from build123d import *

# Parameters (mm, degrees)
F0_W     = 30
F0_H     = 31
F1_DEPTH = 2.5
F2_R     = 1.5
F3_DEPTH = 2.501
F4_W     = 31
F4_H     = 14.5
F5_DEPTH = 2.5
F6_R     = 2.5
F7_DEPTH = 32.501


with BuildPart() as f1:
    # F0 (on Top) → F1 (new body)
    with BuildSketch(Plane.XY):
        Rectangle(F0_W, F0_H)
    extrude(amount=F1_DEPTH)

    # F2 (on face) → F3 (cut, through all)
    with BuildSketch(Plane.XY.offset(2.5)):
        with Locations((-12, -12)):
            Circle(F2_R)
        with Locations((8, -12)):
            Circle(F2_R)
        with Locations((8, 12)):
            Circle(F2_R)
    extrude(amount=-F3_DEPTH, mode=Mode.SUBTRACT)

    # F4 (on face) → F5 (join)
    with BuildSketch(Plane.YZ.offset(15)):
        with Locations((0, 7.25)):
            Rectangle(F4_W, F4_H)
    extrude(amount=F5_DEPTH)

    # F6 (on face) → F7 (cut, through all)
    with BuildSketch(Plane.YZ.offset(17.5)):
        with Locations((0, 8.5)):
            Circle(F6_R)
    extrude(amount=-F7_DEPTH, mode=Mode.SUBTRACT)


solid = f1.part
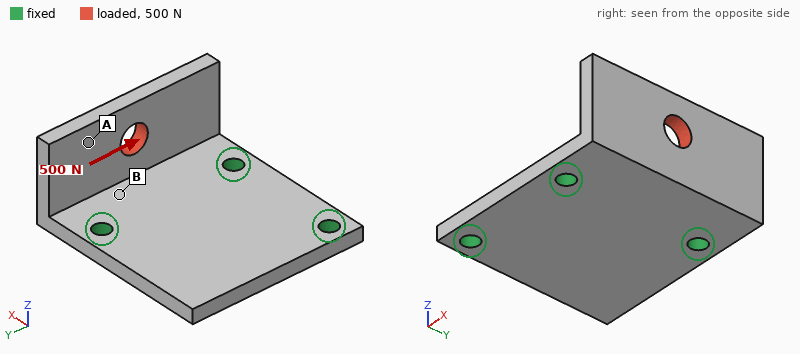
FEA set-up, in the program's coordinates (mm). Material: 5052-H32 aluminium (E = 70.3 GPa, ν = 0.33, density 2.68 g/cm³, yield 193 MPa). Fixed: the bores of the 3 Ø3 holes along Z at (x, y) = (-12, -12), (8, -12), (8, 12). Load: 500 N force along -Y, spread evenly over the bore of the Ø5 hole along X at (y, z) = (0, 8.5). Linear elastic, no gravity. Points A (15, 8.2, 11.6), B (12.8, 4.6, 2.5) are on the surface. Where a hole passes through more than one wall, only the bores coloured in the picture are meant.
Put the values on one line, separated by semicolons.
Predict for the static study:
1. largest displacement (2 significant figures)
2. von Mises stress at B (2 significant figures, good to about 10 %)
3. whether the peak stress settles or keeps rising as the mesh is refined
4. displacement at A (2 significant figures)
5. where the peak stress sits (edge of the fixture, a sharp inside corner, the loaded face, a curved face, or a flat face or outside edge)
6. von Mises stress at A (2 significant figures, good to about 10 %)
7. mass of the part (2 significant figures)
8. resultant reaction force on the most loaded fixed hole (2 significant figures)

35 µm; 33 MPa; keeps rising; 23 µm; edge of the fixture; 12 MPa; 9.0 g; 330 N
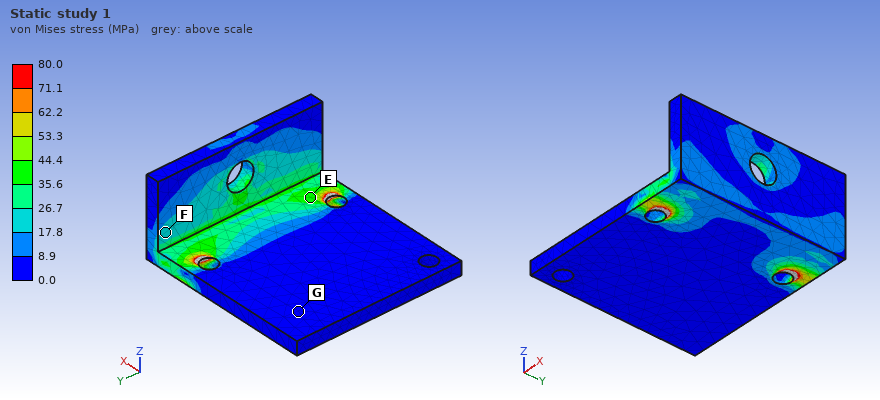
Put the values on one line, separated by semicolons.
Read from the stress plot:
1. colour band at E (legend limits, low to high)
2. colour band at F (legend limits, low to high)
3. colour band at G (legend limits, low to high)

35.6 to 44.4 MPa; 17.8 to 26.7 MPa; 0.0 to 8.9 MPa
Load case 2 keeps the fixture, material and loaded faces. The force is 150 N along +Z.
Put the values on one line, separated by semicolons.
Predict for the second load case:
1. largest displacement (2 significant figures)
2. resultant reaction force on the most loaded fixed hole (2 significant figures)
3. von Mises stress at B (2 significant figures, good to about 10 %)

28 µm; 83 N; 12 MPa
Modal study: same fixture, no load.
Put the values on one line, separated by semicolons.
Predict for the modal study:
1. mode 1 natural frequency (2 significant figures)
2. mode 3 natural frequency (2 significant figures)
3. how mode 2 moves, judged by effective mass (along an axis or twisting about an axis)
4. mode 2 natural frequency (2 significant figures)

5900 Hz; 10 kHz; along Z; 6800 Hz
